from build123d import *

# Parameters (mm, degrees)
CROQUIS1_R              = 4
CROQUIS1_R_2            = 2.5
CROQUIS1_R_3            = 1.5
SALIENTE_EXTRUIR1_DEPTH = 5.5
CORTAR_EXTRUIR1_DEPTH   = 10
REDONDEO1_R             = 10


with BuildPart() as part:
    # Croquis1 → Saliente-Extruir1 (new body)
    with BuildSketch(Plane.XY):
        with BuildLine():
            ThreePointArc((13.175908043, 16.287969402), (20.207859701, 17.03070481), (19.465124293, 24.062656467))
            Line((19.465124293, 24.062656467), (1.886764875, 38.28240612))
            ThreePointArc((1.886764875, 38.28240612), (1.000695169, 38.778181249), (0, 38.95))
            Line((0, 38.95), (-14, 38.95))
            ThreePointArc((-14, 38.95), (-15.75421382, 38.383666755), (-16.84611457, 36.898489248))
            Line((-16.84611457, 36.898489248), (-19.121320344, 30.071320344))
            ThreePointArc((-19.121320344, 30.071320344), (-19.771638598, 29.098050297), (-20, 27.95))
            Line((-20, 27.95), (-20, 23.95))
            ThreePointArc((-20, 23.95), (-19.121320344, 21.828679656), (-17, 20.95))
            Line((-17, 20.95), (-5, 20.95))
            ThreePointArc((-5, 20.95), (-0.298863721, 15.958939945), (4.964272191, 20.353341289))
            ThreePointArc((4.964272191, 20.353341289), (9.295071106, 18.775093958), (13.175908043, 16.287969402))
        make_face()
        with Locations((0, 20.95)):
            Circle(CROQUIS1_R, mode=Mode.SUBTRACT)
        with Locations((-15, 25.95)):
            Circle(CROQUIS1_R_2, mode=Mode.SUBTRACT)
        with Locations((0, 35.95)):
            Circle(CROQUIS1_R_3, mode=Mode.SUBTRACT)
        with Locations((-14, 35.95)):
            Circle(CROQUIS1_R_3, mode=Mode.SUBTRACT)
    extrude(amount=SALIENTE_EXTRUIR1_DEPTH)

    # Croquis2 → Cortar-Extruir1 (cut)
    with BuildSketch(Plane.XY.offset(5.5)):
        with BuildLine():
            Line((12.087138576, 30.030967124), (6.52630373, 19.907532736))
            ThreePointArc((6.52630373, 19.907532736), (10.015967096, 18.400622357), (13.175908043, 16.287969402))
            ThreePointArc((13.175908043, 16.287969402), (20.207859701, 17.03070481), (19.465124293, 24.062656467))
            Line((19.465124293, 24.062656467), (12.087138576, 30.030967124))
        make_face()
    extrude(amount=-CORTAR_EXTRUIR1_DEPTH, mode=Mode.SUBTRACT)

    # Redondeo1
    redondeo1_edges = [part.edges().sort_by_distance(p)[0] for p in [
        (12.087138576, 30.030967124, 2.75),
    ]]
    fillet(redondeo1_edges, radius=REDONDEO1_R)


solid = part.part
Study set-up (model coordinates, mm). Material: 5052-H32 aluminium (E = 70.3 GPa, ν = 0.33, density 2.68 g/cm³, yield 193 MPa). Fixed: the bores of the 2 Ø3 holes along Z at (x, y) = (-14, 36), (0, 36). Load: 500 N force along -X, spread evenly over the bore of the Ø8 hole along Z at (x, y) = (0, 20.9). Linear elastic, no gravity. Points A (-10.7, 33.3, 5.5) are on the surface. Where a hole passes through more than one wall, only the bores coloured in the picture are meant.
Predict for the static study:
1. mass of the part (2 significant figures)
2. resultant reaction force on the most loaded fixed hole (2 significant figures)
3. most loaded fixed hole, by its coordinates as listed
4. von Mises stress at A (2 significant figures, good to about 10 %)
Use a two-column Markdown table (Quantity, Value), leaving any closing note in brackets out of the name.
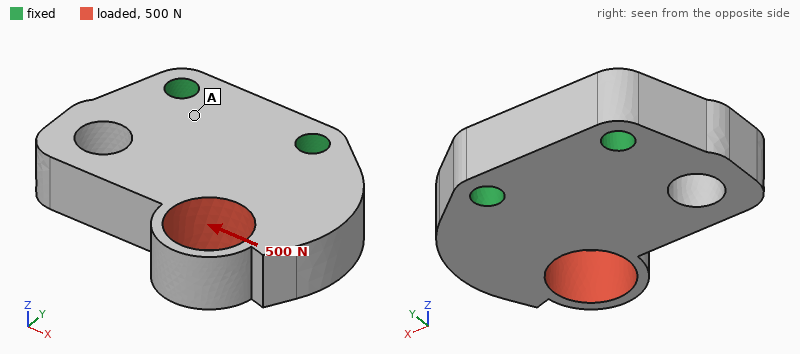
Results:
| Quantity | Value |
|---|---|
| mass of the part | 6.3 g |
| resultant reaction force on the most loaded fixed hole | 550 N |
| most loaded fixed hole, by its coordinates as listed | (-14, 36) |
| von Mises stress at A | 14 MPa |
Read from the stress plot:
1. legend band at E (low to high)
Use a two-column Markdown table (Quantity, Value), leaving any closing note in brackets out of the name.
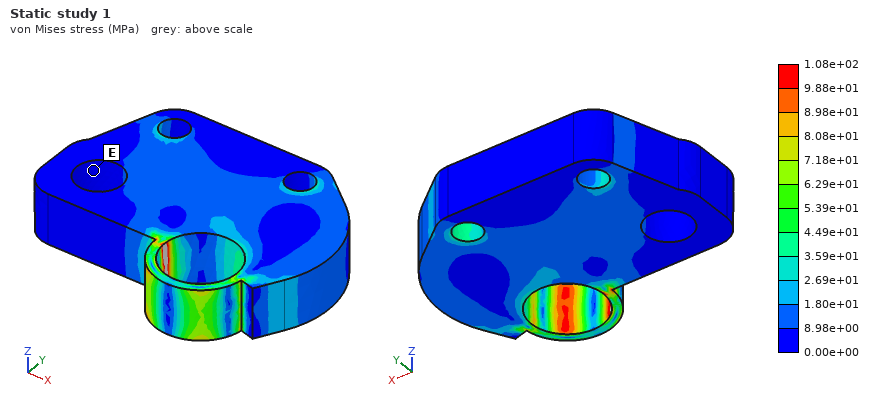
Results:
| Quantity | Value |
|---|---|
| legend band at E | 0.00e+00 to 8.98e+00 MPa |
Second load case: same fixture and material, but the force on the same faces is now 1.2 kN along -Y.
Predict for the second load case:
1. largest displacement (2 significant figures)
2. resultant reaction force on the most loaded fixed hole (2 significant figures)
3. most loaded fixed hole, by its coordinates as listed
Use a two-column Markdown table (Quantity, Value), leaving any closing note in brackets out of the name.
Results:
| Quantity | Value |
|---|---|
| largest displacement | 16 µm |
| resultant reaction force on the most loaded fixed hole | 1.1 kN |
| most loaded fixed hole, by its coordinates as listed | (0, 36) |
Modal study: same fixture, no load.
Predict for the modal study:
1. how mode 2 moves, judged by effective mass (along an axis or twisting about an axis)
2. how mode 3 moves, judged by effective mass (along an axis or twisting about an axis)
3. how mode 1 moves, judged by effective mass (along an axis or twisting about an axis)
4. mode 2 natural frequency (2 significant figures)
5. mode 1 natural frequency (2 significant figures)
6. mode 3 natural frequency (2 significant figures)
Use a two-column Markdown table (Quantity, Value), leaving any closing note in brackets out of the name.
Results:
| Quantity | Value |
|---|---|
| how mode 2 moves, judged by effective mass | twisting about Y |
| how mode 3 moves, judged by effective mass | along X |
| how mode 1 moves, judged by effective mass | along Z |
| mode 2 natural frequency | 23 kHz |
| mode 1 natural frequency | 16 kHz |
| mode 3 natural frequency | 30 kHz |
